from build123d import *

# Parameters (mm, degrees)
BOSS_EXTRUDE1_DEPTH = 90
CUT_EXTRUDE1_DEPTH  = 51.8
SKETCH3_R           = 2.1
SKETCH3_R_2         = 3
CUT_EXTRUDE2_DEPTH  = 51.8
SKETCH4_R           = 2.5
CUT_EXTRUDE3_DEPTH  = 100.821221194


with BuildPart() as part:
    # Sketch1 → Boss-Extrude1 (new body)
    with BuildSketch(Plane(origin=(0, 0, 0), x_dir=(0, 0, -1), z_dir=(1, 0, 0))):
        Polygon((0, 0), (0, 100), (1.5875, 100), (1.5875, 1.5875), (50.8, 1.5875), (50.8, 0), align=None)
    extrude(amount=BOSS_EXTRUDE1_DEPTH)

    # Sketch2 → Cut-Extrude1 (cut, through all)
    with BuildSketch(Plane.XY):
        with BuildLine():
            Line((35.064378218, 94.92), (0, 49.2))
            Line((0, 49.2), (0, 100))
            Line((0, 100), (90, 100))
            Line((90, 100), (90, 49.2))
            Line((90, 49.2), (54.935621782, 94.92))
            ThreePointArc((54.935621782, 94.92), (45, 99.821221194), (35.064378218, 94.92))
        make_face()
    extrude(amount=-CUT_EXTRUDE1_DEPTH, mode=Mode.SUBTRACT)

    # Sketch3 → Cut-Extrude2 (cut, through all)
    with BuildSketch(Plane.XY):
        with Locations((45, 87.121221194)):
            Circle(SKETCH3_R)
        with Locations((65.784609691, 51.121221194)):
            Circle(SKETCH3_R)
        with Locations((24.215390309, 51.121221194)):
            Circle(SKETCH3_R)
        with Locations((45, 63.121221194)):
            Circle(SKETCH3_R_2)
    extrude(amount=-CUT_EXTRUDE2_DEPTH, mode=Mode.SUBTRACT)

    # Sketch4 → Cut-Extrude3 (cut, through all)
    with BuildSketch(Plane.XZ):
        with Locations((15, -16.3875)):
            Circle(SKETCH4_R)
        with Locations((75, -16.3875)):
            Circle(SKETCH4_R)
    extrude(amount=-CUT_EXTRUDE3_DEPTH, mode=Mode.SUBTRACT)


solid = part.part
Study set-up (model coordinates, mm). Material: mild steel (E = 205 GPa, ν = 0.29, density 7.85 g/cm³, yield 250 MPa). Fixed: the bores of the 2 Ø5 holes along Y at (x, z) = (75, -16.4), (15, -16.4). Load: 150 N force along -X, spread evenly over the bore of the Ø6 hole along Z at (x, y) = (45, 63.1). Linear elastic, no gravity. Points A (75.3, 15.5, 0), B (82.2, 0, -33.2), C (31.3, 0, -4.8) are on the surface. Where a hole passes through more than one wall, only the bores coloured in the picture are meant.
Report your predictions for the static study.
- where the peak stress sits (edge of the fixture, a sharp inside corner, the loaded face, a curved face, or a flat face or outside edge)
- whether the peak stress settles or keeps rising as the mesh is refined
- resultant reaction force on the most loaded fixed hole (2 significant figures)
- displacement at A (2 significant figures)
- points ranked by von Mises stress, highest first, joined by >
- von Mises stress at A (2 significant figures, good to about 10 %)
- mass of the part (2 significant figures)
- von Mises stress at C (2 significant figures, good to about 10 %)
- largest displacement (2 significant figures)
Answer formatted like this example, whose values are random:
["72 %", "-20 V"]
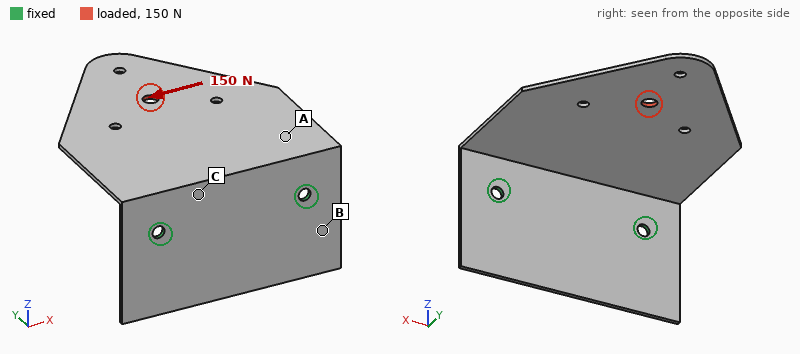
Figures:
["edge of the fixture", "keeps rising", "170 N", "0.075 mm", "C > A > B", "19 MPa", "140 g", "30 MPa", "0.18 mm"]
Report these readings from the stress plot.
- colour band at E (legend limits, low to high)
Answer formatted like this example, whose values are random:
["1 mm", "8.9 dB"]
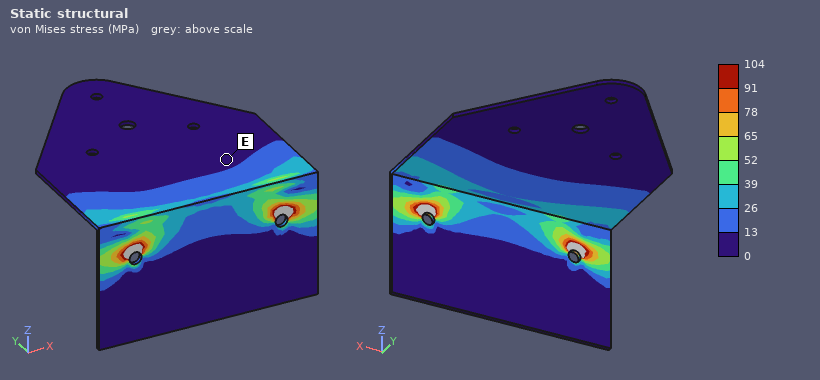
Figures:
["0 to 13 MPa"]
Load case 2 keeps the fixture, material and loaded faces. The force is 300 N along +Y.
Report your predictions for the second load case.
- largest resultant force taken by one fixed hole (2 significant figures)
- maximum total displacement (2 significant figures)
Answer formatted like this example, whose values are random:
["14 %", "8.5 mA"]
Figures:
["150 N", "0.65 mm"]
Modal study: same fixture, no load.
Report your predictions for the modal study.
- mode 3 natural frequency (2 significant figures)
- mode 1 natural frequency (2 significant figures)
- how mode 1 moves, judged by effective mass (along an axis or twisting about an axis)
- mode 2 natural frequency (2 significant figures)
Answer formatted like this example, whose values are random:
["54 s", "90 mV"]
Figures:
["770 Hz", "150 Hz", "along Z", "520 Hz"]
